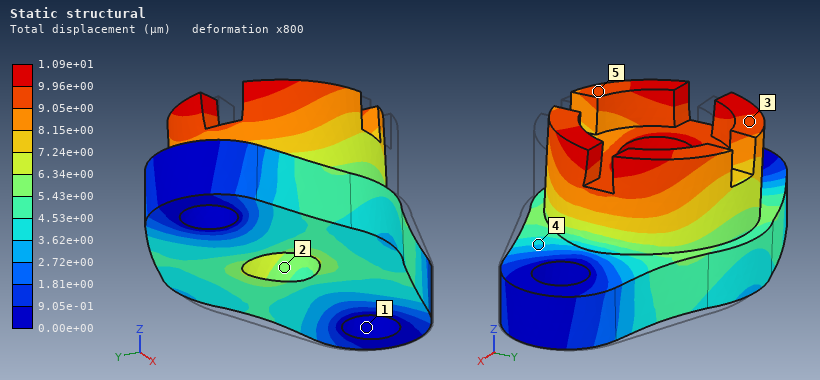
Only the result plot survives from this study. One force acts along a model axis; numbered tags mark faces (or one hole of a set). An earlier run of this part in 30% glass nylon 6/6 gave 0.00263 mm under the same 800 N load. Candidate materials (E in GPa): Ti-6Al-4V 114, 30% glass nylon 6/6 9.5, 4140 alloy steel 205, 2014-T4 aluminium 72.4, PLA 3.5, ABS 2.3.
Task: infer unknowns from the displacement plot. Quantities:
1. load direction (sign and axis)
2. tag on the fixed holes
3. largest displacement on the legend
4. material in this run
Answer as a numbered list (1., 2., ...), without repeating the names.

1. -X
2. 1
3. 1.09e+01 µm
4. ABS
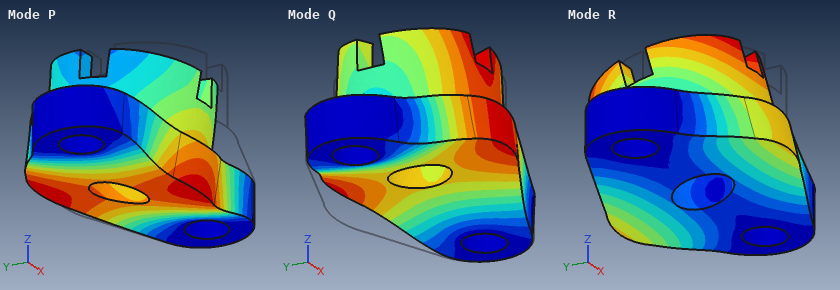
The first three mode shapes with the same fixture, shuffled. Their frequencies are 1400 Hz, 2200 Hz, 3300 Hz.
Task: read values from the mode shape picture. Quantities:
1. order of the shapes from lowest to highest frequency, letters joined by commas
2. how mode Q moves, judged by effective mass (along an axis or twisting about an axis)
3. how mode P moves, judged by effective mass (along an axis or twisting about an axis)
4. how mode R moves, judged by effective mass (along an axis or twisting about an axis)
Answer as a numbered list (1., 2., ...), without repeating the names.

1. R, Q, P
2. along Z
3. along Y
4. along Y
